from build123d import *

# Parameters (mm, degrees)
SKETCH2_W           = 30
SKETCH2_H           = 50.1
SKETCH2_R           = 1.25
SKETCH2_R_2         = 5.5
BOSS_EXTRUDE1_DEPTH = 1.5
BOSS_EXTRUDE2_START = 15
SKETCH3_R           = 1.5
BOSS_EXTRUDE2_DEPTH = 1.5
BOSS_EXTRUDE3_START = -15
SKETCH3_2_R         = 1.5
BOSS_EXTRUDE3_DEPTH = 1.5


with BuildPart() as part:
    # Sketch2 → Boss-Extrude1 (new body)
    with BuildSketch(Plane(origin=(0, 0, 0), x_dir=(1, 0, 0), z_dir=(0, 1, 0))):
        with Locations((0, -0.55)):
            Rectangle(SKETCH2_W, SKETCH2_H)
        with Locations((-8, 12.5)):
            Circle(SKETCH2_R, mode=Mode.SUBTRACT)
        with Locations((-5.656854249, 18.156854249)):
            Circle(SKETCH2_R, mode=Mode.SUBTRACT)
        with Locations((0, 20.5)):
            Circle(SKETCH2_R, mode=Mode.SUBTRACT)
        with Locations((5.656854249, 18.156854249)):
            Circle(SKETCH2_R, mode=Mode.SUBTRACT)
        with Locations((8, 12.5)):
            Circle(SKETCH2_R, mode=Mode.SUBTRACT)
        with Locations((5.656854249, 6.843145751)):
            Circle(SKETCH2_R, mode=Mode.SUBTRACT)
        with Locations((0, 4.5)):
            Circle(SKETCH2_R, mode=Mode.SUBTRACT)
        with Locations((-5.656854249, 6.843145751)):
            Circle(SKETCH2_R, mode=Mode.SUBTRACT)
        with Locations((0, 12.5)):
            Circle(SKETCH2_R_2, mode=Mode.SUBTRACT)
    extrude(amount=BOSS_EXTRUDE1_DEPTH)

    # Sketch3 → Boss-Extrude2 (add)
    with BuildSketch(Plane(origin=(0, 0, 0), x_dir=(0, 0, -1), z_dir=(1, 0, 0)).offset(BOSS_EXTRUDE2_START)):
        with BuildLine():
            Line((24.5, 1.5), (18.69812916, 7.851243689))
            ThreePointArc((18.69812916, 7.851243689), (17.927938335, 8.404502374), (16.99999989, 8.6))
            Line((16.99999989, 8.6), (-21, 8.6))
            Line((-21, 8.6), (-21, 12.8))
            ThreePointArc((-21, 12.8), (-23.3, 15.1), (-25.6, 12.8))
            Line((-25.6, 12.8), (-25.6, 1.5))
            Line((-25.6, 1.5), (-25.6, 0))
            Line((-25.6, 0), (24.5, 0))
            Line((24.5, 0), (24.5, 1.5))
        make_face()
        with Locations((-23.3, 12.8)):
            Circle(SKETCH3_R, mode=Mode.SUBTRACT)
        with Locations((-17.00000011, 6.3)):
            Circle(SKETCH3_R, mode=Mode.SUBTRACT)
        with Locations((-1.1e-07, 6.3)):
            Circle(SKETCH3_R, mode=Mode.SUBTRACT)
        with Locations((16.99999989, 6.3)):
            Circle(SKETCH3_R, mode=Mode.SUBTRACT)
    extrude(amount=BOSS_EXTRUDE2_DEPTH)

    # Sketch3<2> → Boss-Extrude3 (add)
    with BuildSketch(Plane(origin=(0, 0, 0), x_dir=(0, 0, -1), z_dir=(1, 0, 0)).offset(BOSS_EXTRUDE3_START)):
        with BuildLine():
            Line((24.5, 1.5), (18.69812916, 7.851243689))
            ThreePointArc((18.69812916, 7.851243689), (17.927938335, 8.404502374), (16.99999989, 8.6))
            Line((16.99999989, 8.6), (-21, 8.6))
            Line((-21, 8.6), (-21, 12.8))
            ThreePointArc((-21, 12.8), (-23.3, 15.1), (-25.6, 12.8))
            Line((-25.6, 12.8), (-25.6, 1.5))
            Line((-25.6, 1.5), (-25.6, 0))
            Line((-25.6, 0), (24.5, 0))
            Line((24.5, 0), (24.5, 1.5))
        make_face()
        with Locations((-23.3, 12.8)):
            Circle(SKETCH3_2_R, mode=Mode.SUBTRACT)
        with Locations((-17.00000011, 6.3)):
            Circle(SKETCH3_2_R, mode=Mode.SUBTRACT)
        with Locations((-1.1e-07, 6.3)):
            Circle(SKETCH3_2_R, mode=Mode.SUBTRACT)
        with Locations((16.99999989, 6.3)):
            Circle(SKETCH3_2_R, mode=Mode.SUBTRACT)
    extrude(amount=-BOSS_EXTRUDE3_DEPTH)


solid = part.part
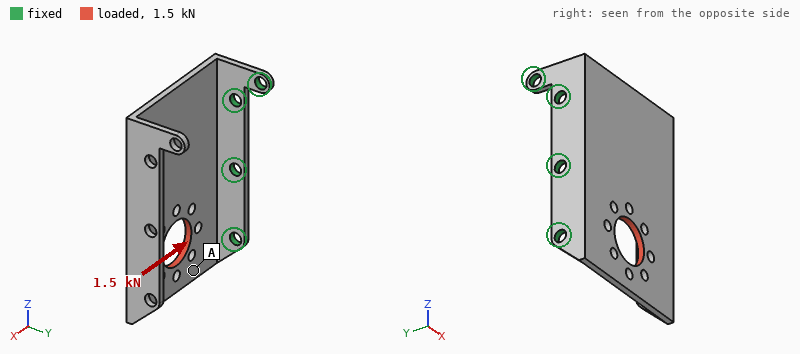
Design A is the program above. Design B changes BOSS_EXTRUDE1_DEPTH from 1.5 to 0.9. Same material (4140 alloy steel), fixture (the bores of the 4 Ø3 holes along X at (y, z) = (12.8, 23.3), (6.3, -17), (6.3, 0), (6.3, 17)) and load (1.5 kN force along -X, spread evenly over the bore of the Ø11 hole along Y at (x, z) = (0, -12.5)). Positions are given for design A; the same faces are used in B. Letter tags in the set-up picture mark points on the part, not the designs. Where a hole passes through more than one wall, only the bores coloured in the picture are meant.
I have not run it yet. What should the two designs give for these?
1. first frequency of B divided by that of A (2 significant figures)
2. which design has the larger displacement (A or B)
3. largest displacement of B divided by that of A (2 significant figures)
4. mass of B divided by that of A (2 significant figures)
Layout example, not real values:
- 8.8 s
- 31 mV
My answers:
- 0.60
- B
- 1.2
- 0.75
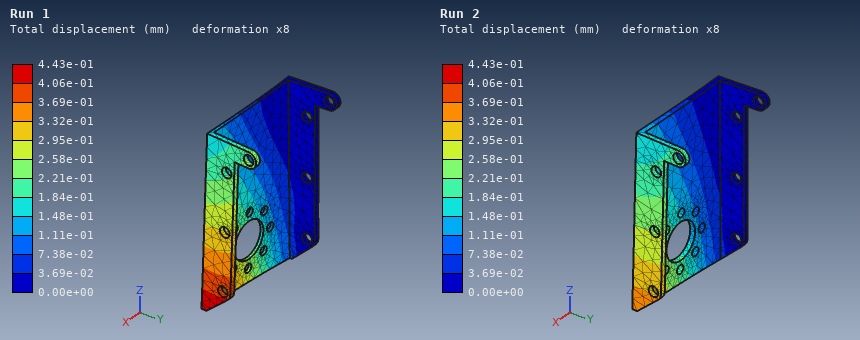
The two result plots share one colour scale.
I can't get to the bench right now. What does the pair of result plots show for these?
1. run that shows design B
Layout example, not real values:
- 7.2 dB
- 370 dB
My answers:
- Run 1
